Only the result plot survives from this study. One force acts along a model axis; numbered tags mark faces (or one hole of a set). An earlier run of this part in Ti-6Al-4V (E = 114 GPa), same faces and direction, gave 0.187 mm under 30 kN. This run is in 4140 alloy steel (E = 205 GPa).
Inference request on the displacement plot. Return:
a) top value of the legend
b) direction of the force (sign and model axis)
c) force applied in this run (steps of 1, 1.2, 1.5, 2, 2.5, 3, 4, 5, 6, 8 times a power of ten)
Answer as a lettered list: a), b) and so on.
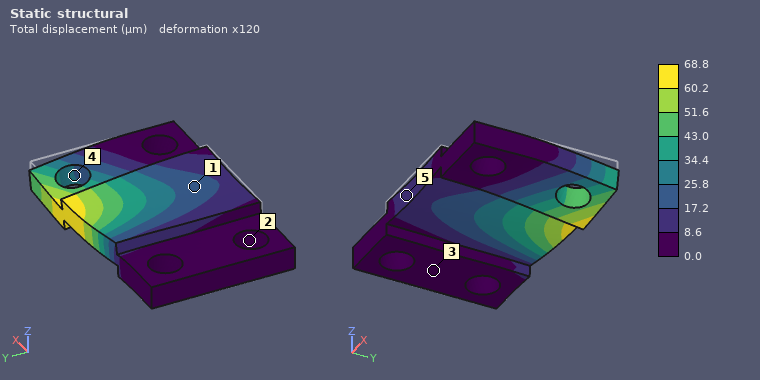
a) 68.8 µm
b) -Z
c) 20 kN
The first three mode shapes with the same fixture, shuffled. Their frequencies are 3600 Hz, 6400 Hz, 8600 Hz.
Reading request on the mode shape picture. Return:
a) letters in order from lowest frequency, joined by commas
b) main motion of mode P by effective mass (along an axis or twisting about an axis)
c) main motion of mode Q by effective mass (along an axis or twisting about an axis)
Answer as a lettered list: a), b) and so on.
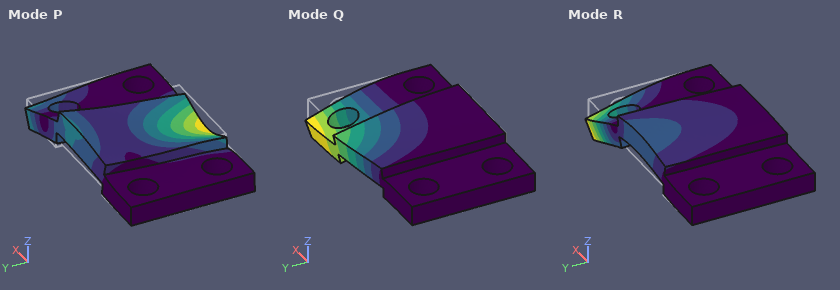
a) Q, R, P
b) along Z
c) along Z
